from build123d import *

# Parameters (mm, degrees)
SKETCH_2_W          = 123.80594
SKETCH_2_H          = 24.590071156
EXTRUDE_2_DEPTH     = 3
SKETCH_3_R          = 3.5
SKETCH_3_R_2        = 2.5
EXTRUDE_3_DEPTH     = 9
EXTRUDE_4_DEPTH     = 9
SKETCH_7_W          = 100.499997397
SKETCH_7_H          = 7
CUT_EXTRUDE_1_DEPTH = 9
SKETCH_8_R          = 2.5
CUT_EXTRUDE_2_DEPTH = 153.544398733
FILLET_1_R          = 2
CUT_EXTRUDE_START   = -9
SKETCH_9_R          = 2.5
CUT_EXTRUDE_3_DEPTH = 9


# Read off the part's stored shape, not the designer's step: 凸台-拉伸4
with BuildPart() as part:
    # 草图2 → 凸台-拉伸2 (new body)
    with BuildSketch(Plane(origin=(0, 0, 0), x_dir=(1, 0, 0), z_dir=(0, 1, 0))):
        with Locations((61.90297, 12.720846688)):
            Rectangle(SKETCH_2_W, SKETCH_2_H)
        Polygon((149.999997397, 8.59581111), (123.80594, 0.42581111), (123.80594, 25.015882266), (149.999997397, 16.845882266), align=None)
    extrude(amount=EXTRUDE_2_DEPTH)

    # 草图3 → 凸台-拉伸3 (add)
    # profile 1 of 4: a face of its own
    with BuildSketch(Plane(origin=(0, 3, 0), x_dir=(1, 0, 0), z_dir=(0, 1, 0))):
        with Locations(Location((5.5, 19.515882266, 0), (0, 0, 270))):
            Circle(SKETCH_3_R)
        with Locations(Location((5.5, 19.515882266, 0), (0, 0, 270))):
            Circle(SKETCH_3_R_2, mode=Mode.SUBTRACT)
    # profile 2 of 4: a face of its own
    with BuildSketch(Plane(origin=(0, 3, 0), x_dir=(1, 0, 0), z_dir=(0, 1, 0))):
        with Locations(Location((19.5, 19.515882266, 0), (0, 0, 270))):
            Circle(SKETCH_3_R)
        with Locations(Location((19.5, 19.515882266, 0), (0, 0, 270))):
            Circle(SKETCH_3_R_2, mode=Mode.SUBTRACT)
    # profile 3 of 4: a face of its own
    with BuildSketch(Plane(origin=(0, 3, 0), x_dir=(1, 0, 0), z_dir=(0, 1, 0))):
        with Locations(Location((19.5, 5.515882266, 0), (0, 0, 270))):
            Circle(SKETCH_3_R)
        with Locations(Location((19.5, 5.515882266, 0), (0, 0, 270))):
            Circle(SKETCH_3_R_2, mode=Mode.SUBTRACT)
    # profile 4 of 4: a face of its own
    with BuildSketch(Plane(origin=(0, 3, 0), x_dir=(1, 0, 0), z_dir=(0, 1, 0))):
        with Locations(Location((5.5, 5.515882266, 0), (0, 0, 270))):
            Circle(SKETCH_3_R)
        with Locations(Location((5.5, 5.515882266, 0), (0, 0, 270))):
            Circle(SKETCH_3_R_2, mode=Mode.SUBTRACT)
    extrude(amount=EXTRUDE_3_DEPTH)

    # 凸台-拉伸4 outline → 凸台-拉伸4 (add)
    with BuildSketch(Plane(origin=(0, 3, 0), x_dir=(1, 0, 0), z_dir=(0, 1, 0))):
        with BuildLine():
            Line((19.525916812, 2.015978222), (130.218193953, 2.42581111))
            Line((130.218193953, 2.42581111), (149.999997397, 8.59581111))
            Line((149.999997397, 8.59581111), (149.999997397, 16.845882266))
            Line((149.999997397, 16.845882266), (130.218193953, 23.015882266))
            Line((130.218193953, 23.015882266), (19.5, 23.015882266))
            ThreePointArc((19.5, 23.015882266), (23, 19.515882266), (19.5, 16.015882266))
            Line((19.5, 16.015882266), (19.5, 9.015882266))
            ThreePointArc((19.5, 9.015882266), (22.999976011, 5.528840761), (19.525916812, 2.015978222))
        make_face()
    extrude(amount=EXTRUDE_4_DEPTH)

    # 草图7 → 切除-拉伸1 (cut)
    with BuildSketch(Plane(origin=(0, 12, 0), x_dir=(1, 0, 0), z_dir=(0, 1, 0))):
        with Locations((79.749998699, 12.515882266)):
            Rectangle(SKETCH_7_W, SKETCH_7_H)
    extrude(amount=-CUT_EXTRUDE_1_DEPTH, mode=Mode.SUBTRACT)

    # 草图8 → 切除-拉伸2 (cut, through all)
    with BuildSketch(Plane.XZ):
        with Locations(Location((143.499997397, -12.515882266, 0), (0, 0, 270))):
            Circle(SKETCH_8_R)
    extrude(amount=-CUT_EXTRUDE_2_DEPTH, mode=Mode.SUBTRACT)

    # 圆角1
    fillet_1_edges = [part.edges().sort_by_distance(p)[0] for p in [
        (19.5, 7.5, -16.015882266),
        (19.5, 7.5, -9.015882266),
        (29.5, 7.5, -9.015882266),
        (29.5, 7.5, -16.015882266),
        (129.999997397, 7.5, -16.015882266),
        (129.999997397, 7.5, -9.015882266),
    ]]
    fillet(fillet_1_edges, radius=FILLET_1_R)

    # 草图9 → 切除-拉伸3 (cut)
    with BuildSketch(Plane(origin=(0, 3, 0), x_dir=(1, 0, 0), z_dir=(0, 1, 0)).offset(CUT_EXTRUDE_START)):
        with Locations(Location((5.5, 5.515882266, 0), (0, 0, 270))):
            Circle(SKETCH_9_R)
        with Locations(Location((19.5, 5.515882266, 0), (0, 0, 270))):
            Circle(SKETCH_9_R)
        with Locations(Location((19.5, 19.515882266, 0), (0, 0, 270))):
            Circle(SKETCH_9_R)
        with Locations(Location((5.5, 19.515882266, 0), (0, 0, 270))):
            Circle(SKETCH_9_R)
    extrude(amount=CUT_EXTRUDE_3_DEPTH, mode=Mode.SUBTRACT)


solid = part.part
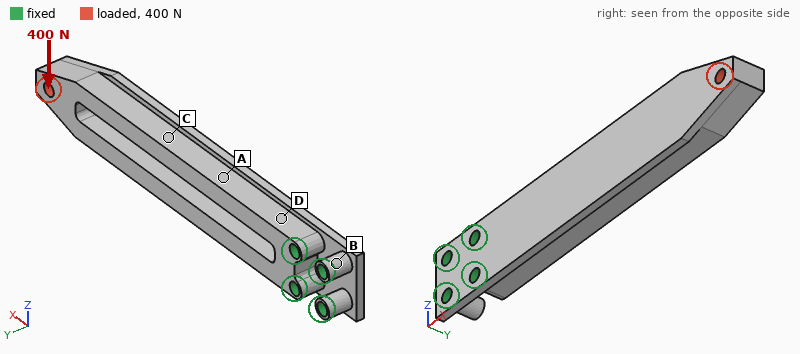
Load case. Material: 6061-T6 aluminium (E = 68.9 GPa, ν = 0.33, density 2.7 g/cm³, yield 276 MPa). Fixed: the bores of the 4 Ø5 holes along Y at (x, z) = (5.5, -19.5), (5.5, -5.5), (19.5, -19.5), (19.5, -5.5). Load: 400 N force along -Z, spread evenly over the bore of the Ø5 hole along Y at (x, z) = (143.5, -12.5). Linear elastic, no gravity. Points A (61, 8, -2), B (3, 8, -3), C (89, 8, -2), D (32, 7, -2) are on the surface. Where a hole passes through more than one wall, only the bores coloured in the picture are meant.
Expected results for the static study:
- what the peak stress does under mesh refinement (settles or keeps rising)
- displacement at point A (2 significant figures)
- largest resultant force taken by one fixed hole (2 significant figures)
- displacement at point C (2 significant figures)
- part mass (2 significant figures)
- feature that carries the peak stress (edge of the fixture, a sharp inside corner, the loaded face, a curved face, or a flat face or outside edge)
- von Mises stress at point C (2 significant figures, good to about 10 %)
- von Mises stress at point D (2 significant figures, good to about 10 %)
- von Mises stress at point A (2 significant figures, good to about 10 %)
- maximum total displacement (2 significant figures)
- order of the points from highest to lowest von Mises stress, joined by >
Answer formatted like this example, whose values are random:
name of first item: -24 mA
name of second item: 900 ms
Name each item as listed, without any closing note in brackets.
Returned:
what the peak stress does under mesh refinement: keeps rising
displacement at point A: 0.072 mm
largest resultant force taken by one fixed hole: 3.1 kN
displacement at point C: 0.17 mm
part mass: 74 g
feature that carries the peak stress: edge of the fixture
von Mises stress at point C: 25 MPa
von Mises stress at point D: 50 MPa
von Mises stress at point A: 35 MPa
maximum total displacement: 0.45 mm
order of the points from highest to lowest von Mises stress, joined by >: D > A > C > B
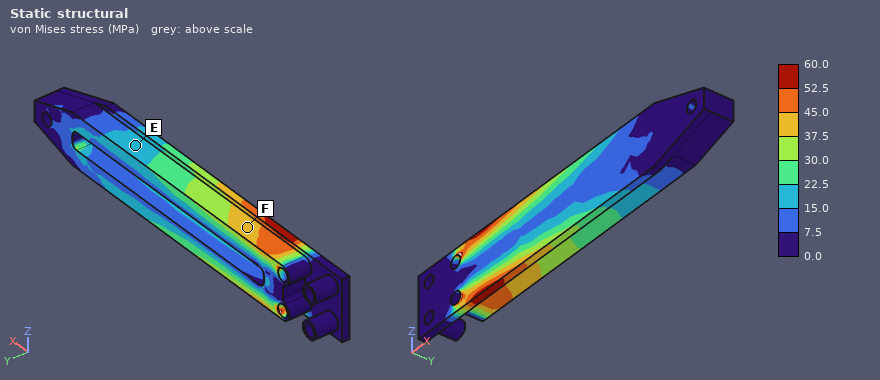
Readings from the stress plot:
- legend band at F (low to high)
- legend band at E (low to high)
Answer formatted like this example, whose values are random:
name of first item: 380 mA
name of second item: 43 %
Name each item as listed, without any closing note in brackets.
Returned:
legend band at F: 37.5 to 45.0 MPa
legend band at E: 15.0 to 22.5 MPa
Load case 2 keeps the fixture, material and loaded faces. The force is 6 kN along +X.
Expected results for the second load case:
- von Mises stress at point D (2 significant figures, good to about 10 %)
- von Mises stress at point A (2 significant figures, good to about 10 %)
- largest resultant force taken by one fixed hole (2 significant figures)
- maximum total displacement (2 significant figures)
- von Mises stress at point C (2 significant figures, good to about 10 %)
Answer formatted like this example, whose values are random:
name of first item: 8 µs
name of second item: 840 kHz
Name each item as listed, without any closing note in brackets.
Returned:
von Mises stress at point D: 31 MPa
von Mises stress at point A: 35 MPa
largest resultant force taken by one fixed hole: 3.0 kN
maximum total displacement: 0.21 mm
von Mises stress at point C: 36 MPa
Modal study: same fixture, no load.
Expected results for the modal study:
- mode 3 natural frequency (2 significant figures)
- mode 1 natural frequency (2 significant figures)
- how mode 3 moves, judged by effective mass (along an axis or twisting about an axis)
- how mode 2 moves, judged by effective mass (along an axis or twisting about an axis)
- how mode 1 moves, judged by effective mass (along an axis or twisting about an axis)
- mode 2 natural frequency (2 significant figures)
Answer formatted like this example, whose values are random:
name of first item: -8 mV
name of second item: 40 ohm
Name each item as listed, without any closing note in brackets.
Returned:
mode 3 natural frequency: 3200 Hz
mode 1 natural frequency: 650 Hz
how mode 3 moves, judged by effective mass: twisting about X
how mode 2 moves, judged by effective mass: along Z
how mode 1 moves, judged by effective mass: along Y
mode 2 natural frequency: 1200 Hz
